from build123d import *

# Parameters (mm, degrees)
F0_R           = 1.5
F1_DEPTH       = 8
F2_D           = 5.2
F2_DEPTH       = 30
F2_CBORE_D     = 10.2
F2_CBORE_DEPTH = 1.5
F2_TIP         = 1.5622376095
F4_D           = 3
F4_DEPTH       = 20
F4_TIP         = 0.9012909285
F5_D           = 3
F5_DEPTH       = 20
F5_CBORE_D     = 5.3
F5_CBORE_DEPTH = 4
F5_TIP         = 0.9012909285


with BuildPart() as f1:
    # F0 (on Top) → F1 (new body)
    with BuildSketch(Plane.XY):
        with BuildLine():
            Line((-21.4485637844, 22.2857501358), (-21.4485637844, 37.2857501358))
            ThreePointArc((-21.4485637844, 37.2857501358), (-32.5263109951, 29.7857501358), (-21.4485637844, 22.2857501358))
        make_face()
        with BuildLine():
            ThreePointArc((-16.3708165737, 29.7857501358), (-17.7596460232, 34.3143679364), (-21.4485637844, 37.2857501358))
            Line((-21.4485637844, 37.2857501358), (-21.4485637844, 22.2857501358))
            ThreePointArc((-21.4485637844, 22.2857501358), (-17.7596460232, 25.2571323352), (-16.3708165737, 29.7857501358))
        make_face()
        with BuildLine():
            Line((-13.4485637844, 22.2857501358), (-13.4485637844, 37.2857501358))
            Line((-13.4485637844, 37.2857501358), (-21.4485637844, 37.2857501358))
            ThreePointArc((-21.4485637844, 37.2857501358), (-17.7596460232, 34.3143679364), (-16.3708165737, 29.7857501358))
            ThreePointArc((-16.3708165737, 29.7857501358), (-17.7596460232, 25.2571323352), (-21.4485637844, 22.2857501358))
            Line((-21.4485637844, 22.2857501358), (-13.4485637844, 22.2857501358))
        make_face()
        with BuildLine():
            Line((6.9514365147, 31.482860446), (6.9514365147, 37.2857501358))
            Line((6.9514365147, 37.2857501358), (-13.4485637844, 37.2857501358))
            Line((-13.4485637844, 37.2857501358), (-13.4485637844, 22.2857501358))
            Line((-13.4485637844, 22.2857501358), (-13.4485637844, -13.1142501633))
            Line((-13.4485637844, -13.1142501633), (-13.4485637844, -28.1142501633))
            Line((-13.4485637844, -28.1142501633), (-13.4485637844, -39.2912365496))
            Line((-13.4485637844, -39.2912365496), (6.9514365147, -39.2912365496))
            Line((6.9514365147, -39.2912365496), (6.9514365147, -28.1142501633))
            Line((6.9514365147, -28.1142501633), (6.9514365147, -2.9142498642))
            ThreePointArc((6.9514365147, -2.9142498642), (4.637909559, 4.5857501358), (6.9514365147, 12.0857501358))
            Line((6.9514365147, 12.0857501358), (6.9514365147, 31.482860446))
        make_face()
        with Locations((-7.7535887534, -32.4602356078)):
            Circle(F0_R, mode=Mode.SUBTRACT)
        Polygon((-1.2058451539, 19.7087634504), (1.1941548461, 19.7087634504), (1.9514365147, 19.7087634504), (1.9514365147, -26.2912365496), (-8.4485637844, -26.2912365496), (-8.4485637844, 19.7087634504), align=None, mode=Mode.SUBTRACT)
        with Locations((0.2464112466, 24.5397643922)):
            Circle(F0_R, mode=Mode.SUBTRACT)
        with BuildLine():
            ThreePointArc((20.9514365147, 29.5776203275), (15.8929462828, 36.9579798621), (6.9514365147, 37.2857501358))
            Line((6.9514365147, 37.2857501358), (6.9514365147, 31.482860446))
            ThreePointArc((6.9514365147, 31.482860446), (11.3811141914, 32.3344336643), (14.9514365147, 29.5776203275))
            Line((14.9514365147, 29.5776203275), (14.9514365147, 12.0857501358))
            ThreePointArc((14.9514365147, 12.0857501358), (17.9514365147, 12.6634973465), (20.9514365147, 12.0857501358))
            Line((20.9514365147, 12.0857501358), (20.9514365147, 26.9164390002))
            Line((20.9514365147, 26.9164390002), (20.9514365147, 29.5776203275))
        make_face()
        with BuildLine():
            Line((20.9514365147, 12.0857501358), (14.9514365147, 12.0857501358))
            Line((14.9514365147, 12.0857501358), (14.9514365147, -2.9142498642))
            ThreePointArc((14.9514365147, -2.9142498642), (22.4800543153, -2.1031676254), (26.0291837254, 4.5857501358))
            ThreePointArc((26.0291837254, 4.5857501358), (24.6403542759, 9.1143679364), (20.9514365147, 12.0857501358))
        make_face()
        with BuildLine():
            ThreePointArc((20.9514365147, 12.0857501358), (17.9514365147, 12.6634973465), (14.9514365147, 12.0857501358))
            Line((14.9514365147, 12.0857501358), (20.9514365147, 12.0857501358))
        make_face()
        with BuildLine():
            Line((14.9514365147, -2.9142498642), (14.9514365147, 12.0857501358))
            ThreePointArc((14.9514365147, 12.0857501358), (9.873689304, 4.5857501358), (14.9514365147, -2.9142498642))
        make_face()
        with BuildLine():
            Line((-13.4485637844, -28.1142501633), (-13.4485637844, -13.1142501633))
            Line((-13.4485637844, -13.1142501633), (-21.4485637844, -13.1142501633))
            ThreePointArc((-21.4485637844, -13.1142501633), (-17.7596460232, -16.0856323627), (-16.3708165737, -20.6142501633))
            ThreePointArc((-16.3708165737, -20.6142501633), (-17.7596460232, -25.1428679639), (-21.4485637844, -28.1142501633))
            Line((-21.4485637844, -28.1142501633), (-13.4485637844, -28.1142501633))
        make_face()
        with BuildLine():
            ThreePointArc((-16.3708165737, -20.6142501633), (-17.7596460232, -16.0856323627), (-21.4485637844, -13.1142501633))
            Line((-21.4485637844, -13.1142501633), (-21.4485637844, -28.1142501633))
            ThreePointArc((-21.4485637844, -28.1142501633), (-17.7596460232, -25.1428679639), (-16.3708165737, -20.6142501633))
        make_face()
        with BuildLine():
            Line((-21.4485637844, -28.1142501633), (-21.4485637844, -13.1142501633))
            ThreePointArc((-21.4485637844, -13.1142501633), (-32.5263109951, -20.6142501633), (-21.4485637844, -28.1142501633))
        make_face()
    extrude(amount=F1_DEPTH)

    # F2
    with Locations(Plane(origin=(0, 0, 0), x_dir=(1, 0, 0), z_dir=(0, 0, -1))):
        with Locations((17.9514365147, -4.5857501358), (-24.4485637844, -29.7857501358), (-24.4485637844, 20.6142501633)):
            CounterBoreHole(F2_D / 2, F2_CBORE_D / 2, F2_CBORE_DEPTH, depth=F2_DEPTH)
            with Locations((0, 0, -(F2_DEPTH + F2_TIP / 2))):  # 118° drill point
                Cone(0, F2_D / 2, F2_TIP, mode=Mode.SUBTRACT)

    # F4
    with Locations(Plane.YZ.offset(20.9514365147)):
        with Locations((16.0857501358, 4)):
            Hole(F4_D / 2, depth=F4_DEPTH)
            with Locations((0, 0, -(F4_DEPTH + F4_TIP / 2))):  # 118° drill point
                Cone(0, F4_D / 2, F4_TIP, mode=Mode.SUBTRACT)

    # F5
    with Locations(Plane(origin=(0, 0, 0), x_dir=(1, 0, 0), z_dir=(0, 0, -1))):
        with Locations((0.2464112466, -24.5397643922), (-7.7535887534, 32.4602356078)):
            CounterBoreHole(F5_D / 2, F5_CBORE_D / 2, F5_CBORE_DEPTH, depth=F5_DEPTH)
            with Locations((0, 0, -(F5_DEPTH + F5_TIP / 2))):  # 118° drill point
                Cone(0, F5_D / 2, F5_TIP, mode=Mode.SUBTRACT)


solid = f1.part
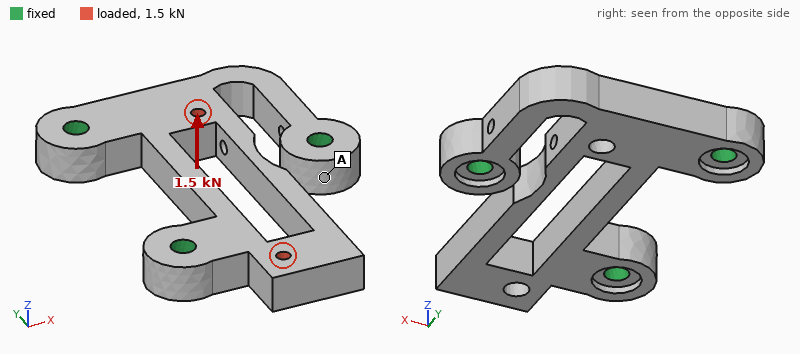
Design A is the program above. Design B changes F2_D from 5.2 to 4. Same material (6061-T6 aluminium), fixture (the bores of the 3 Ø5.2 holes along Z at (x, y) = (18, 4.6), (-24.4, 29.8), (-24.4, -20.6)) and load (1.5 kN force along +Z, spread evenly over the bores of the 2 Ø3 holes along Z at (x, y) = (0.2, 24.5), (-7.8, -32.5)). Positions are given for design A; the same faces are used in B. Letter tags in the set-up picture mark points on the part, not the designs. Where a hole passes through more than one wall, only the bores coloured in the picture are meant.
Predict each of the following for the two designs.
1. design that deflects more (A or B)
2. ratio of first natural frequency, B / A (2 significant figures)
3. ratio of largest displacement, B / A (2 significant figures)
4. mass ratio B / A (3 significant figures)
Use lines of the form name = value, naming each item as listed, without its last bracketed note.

design that deflects more = B
ratio of first natural frequency, B / A = 0.96
ratio of largest displacement, B / A = 1.1
mass ratio B / A = 1.01
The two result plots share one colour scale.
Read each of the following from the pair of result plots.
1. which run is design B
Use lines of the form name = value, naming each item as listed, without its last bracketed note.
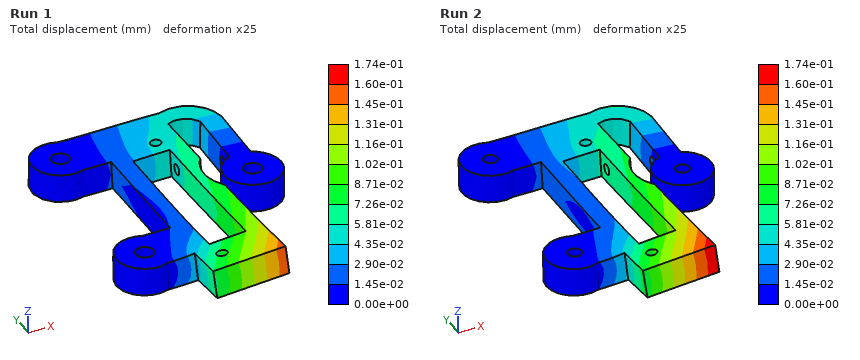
which run is design B = Run 2
